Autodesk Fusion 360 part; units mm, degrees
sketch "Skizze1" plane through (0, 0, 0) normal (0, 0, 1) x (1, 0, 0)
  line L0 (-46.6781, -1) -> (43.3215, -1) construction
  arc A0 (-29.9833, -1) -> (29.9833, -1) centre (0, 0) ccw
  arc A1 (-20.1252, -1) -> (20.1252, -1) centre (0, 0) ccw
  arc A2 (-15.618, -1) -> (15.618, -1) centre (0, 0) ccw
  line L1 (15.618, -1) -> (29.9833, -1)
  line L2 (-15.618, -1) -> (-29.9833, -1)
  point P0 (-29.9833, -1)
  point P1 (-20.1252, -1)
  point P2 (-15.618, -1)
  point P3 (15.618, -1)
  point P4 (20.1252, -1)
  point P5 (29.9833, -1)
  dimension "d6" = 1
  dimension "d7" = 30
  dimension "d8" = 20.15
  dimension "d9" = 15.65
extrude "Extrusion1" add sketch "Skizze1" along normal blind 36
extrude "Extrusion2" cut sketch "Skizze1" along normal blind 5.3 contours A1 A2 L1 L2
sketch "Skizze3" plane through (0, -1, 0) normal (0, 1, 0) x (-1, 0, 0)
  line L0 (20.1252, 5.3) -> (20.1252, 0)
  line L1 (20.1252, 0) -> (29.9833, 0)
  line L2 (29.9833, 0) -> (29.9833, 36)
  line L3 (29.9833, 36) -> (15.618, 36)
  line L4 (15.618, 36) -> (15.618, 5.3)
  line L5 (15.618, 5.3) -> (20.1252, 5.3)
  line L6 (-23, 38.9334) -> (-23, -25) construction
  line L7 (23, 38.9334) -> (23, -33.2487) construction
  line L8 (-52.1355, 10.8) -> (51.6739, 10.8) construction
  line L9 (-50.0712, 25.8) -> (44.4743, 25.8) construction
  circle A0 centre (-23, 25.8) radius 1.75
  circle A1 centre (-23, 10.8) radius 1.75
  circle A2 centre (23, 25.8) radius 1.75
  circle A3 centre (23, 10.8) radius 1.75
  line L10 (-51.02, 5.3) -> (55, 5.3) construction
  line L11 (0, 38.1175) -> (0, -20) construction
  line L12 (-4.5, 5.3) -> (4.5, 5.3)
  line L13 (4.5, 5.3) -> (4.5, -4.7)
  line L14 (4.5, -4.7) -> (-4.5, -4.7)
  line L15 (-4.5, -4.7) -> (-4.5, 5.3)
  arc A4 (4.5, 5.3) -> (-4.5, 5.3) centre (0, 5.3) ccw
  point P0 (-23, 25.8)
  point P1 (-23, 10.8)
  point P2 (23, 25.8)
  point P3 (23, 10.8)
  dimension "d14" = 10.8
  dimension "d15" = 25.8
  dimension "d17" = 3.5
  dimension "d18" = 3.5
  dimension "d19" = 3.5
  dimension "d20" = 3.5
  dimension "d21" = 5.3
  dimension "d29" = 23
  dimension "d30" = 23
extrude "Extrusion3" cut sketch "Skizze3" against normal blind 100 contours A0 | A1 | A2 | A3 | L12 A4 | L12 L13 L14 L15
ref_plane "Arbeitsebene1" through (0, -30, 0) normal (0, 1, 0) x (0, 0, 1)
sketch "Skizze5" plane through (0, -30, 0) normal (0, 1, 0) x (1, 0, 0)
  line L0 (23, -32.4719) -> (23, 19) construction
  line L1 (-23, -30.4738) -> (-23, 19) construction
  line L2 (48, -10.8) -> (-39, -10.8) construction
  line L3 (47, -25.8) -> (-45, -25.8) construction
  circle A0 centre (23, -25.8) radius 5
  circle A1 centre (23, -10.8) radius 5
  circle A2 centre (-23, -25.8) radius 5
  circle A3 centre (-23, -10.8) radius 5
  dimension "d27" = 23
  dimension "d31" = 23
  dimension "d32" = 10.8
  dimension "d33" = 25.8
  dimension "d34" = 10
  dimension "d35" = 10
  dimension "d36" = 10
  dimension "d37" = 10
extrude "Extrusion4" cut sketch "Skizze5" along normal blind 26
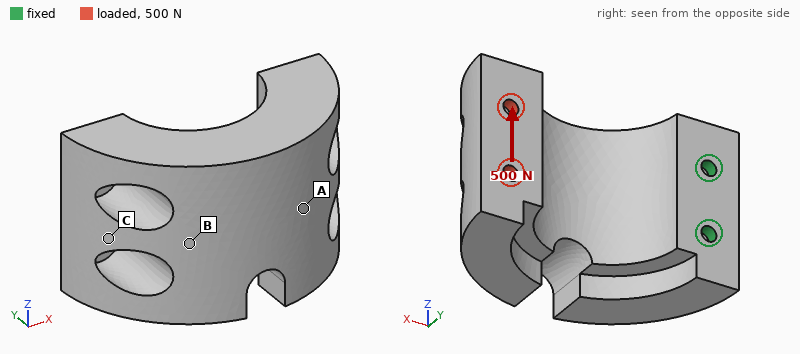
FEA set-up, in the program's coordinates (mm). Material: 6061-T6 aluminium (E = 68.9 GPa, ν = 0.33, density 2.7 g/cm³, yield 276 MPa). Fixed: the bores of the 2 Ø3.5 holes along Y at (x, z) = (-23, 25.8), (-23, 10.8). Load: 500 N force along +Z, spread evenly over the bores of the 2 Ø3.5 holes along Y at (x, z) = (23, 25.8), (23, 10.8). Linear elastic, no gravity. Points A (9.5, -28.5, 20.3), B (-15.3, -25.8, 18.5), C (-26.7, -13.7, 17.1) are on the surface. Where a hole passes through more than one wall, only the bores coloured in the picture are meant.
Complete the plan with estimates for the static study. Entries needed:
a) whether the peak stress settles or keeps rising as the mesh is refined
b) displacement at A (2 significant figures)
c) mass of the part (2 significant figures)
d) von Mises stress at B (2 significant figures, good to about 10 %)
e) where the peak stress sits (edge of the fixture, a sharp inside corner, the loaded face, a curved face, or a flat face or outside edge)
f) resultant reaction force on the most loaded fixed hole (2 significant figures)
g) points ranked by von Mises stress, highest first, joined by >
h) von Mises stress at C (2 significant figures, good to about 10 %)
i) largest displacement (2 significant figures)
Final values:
keeps rising
0.034 mm
78 g
13 MPa
edge of the fixture
1.3 kN
C > B > A
24 MPa
0.11 mm
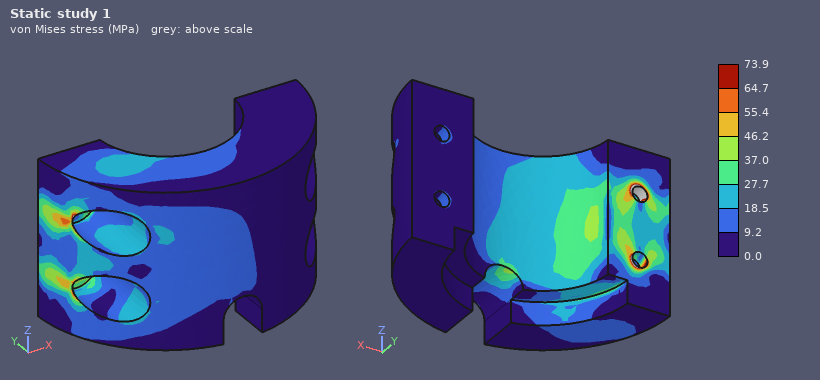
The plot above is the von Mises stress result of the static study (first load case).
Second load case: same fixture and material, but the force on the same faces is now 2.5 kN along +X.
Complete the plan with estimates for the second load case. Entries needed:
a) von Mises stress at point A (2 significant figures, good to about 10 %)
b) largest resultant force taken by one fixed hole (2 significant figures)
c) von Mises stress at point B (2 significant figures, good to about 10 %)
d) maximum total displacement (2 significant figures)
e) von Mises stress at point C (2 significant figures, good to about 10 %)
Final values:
33 MPa
1.3 kN
30 MPa
0.17 mm
21 MPa
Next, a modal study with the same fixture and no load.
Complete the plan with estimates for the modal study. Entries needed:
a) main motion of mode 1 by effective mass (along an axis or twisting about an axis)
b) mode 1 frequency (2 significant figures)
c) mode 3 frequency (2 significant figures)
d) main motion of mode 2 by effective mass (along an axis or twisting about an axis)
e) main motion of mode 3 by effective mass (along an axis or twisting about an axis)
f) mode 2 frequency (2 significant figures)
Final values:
along Y
1000 Hz
4300 Hz
along Z
along Z
2500 Hz
